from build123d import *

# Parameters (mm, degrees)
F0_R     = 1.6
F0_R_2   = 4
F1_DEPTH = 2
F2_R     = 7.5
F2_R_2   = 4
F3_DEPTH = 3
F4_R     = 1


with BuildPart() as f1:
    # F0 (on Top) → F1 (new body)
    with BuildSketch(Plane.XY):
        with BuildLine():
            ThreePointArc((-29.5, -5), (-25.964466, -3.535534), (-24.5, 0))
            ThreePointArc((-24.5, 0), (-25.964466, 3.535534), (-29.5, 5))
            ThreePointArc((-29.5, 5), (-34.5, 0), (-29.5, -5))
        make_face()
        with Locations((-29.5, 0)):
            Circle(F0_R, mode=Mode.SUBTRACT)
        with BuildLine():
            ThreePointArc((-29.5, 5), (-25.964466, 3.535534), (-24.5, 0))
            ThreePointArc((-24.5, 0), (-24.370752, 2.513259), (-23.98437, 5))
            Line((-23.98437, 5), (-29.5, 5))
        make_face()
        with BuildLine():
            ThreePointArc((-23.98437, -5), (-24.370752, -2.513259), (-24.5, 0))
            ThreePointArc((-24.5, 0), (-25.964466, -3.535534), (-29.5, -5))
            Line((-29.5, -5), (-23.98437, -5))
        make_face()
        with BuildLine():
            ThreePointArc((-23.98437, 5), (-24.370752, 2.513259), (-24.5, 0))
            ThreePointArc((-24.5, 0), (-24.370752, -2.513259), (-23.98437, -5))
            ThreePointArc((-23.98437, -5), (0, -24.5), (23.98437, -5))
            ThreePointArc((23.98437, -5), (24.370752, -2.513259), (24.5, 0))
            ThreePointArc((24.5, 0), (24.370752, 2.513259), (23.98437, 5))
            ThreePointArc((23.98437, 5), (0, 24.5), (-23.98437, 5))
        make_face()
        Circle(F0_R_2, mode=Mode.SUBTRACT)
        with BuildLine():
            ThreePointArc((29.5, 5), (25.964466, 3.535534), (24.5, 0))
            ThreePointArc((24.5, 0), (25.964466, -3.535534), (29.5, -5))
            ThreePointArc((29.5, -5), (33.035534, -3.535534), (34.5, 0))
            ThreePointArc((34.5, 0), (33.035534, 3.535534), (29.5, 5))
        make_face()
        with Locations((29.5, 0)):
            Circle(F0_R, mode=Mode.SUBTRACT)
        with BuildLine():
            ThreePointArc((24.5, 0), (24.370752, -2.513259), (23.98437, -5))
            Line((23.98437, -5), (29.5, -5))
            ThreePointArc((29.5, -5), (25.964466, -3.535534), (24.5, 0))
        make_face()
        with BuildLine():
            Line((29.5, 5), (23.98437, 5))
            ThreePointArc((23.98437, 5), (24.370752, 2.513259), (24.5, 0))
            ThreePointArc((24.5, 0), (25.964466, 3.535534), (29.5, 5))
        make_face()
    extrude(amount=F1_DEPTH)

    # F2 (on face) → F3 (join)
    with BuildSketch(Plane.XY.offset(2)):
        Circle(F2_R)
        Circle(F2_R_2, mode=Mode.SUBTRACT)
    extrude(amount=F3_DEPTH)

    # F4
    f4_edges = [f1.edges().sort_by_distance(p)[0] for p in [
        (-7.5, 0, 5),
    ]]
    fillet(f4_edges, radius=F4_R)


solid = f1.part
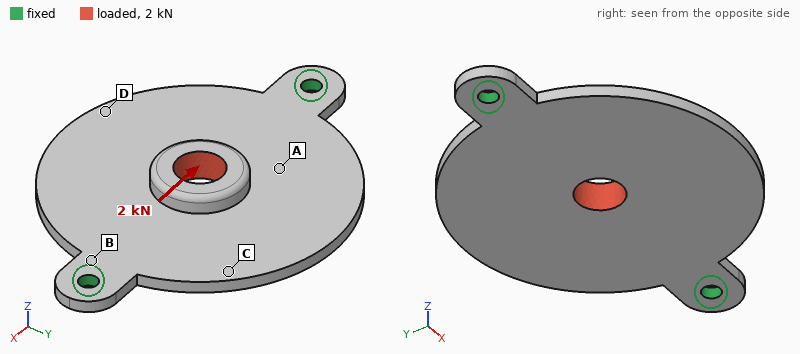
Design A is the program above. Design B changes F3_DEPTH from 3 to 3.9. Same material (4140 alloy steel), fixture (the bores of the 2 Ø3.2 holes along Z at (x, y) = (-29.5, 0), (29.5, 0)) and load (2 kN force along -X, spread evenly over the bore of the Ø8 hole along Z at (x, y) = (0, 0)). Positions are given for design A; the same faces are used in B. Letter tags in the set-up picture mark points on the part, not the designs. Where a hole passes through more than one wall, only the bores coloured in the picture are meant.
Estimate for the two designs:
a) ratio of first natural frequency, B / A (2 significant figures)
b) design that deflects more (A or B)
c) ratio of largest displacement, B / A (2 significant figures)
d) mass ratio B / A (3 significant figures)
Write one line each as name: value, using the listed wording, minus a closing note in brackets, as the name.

ratio of first natural frequency, B / A: 1.00
design that deflects more: B
ratio of largest displacement, B / A: 1.3
mass ratio B / A: 1.03
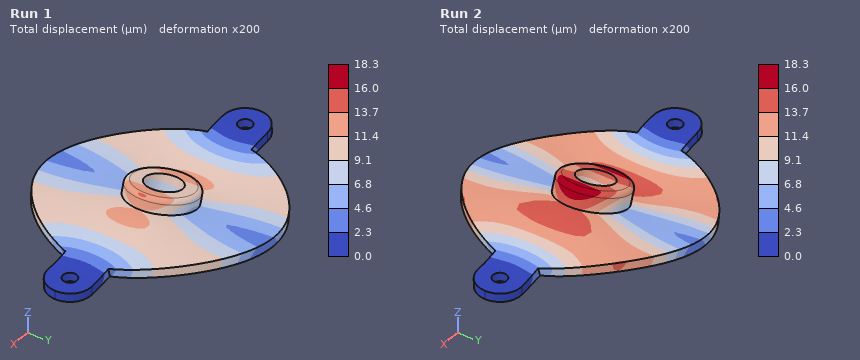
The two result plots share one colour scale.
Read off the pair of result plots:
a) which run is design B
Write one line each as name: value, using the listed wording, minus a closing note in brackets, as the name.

which run is design B: Run 2
